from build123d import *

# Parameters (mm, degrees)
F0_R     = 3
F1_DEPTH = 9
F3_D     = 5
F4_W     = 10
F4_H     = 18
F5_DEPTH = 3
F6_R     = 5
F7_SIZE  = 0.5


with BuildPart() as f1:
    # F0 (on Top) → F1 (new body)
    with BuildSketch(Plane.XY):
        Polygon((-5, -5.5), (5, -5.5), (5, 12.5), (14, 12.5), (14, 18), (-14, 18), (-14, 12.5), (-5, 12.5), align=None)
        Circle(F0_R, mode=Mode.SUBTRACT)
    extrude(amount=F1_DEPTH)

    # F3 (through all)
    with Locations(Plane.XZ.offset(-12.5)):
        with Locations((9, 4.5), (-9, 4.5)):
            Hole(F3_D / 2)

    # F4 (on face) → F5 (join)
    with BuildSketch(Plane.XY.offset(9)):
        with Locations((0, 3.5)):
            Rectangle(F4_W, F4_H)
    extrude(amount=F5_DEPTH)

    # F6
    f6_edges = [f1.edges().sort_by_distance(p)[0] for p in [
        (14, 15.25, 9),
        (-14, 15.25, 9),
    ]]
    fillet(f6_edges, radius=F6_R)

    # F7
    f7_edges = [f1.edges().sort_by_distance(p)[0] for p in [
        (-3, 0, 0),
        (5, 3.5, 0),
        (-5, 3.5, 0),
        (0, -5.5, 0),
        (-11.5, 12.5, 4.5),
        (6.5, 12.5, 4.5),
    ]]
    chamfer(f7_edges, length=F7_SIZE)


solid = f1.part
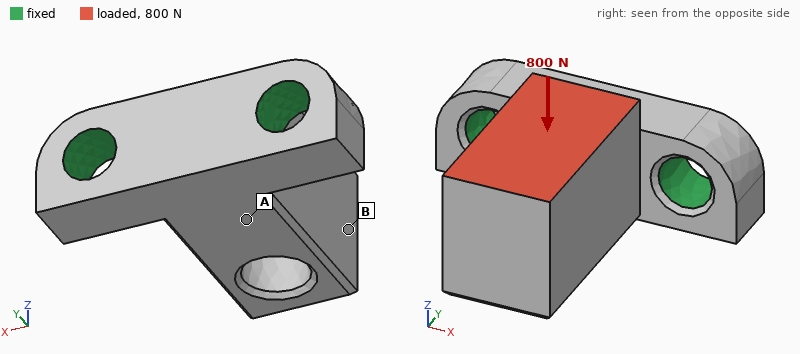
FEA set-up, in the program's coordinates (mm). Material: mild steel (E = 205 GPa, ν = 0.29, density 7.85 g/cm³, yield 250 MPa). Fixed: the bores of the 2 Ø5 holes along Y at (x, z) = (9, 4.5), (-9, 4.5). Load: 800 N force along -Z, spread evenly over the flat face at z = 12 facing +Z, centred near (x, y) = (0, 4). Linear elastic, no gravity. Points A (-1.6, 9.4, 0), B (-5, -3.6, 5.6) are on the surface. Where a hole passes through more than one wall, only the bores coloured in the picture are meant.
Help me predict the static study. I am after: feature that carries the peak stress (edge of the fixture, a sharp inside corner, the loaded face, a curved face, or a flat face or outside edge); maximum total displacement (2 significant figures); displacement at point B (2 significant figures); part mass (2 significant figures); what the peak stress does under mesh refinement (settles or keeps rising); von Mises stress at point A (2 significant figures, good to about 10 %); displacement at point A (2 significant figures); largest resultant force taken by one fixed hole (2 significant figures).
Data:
edge of the fixture
22 µm
19 µm
24 g
keeps rising
27 MPa
6.6 µm
400 N
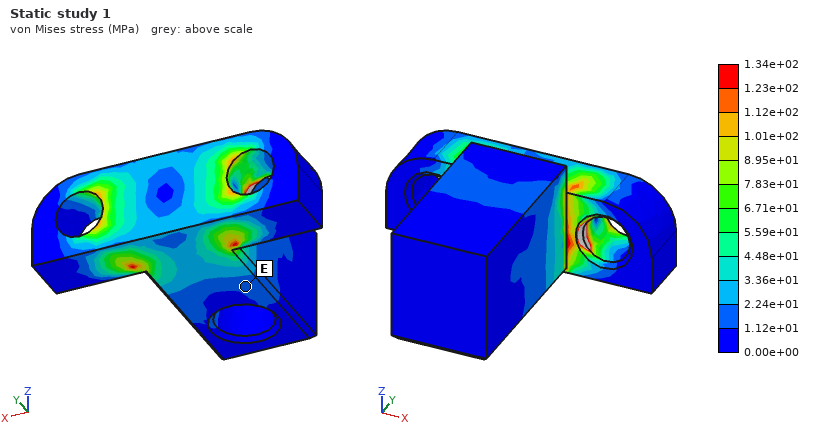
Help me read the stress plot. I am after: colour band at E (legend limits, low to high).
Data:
1.12e+01 to 2.24e+01 MPa
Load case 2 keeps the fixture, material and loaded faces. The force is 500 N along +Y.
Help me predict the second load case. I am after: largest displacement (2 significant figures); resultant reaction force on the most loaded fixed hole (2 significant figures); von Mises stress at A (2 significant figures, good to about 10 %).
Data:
9.3 µm
270 N
12 MPa
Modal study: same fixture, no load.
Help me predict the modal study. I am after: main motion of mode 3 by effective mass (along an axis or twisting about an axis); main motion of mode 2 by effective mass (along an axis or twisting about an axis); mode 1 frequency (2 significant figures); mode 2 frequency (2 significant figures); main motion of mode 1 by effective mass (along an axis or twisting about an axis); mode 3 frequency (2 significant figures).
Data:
twisting about Y
along X
9800 Hz
15 kHz
along Z
33 kHz
